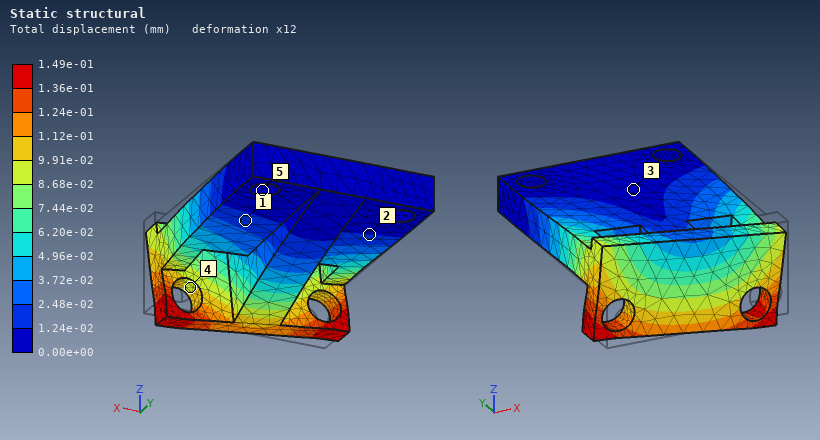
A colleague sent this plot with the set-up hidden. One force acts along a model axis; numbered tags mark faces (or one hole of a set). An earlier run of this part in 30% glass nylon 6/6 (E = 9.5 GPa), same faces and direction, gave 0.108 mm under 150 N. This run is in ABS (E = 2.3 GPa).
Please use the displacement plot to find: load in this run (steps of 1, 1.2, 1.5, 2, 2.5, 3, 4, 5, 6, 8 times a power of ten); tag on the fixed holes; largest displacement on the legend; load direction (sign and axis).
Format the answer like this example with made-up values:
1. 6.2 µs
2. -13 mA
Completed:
1. 50 N
2. 5
3. 1.49e-01 mm
4. -X
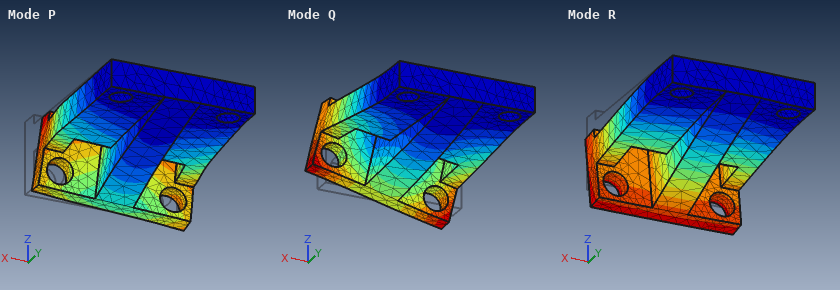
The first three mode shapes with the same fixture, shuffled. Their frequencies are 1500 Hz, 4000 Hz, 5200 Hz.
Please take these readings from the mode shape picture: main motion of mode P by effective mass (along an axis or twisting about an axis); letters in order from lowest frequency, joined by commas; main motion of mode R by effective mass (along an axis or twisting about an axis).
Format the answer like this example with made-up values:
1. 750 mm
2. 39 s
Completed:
1. along X
2. R, Q, P
3. along Z
